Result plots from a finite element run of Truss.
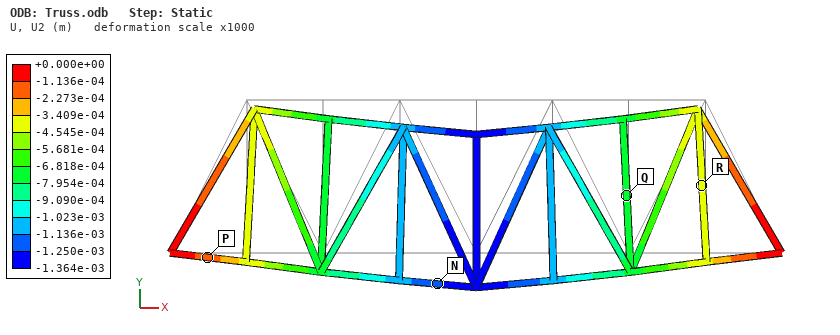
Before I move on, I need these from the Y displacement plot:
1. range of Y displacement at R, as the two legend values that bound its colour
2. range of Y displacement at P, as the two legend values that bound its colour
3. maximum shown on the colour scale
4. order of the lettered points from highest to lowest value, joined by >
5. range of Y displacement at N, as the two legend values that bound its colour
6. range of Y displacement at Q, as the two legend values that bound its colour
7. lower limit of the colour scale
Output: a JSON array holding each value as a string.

["-4.545e-04 to -3.409e-04 m", "-2.273e-04 to -1.136e-04 m", "+0.000e+00 m", "P > R > Q > N", "-1.250e-03 to -1.136e-03 m", "-7.954e-04 to -6.818e-04 m", "-1.364e-03 m"]
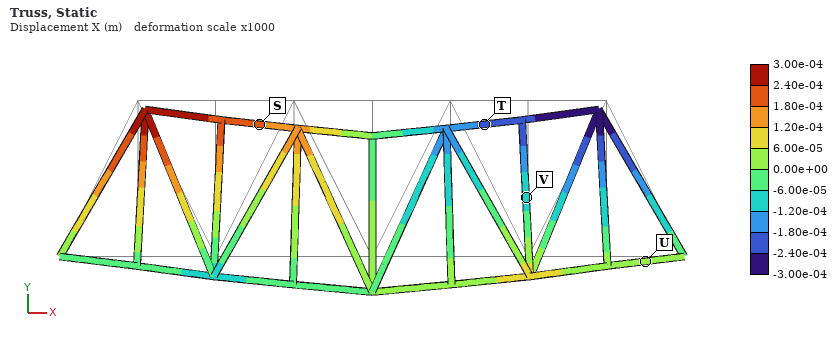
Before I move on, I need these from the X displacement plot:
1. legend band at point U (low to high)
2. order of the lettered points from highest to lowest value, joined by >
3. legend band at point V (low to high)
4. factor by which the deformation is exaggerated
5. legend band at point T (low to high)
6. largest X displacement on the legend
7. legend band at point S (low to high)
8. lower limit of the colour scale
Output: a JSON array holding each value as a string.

["0.00e+00 to 6.00e-05 m", "S > U > V > T", "-1.20e-04 to -6.00e-05 m", "1000", "-2.40e-04 to -1.80e-04 m", "3.00e-04 m", "1.80e-04 to 2.40e-04 m", "-3.00e-04 m"]
